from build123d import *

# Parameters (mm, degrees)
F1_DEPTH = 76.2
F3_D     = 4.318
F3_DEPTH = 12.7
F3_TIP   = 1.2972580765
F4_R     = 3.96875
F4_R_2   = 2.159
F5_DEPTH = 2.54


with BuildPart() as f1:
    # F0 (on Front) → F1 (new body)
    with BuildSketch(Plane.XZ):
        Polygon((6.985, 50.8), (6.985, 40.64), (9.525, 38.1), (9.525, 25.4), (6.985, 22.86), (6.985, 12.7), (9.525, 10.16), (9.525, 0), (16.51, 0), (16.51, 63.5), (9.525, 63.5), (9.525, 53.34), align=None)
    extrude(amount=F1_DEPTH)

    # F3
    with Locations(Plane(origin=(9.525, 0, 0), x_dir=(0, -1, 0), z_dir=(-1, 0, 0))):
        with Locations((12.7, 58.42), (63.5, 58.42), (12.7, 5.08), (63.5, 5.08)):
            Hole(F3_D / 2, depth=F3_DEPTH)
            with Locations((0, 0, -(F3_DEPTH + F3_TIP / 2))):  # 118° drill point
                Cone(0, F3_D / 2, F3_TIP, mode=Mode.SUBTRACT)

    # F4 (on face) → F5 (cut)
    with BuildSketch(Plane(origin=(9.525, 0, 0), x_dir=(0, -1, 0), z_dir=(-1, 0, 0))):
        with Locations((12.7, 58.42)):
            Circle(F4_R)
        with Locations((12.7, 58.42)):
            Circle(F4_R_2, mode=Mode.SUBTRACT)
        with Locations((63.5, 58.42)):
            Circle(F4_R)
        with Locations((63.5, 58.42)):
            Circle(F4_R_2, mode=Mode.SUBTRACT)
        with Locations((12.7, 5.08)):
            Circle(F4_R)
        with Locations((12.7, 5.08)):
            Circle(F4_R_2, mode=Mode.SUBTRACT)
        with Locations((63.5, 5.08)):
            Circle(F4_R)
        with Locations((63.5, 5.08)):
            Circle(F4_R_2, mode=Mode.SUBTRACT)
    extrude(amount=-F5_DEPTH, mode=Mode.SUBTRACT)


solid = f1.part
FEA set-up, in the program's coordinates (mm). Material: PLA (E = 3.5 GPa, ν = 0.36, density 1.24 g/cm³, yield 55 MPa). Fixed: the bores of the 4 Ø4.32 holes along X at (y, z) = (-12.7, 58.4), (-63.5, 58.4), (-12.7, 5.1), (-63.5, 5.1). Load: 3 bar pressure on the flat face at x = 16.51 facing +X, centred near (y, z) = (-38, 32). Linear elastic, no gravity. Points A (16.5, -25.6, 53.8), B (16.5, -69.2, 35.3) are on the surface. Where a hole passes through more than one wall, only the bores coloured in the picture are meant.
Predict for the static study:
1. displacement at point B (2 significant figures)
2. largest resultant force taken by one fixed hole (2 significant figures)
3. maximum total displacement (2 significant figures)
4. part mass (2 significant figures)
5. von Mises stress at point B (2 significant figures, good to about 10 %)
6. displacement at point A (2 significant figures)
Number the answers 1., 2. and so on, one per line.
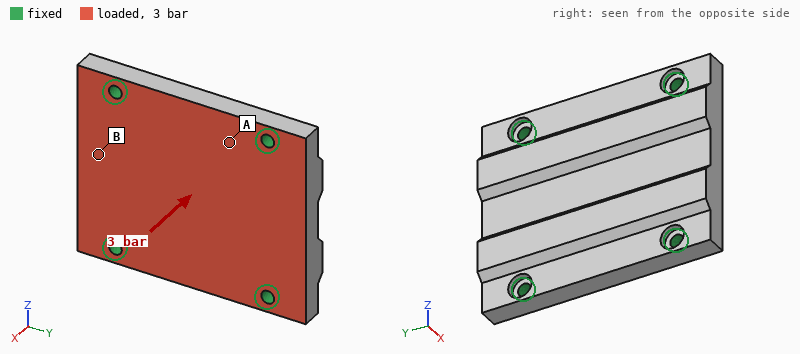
1. 0.13 mm
2. 410 N
3. 0.18 mm
4. 47 g
5. 5.8 MPa
6. 0.083 mm
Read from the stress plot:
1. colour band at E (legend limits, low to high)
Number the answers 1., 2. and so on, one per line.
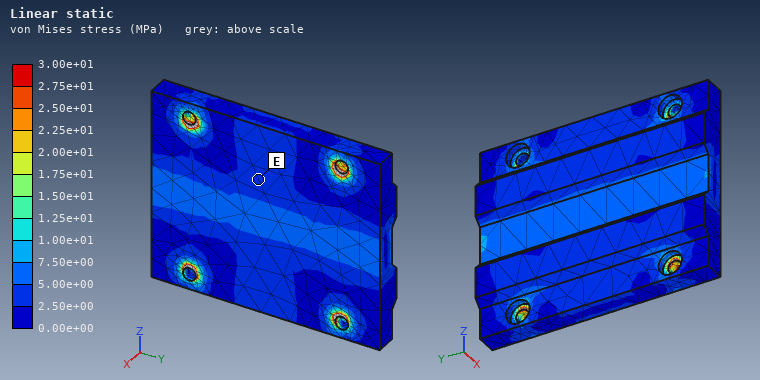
1. 2.50e+00 to 5.00e+00 MPa
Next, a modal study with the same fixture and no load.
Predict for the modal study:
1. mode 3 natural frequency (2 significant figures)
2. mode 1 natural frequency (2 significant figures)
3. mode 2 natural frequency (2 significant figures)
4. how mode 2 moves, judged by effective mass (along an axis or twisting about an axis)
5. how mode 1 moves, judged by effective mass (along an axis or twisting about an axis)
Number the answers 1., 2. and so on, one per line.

1. 3500 Hz
2. 2500 Hz
3. 3200 Hz
4. twisting about Z
5. along X
